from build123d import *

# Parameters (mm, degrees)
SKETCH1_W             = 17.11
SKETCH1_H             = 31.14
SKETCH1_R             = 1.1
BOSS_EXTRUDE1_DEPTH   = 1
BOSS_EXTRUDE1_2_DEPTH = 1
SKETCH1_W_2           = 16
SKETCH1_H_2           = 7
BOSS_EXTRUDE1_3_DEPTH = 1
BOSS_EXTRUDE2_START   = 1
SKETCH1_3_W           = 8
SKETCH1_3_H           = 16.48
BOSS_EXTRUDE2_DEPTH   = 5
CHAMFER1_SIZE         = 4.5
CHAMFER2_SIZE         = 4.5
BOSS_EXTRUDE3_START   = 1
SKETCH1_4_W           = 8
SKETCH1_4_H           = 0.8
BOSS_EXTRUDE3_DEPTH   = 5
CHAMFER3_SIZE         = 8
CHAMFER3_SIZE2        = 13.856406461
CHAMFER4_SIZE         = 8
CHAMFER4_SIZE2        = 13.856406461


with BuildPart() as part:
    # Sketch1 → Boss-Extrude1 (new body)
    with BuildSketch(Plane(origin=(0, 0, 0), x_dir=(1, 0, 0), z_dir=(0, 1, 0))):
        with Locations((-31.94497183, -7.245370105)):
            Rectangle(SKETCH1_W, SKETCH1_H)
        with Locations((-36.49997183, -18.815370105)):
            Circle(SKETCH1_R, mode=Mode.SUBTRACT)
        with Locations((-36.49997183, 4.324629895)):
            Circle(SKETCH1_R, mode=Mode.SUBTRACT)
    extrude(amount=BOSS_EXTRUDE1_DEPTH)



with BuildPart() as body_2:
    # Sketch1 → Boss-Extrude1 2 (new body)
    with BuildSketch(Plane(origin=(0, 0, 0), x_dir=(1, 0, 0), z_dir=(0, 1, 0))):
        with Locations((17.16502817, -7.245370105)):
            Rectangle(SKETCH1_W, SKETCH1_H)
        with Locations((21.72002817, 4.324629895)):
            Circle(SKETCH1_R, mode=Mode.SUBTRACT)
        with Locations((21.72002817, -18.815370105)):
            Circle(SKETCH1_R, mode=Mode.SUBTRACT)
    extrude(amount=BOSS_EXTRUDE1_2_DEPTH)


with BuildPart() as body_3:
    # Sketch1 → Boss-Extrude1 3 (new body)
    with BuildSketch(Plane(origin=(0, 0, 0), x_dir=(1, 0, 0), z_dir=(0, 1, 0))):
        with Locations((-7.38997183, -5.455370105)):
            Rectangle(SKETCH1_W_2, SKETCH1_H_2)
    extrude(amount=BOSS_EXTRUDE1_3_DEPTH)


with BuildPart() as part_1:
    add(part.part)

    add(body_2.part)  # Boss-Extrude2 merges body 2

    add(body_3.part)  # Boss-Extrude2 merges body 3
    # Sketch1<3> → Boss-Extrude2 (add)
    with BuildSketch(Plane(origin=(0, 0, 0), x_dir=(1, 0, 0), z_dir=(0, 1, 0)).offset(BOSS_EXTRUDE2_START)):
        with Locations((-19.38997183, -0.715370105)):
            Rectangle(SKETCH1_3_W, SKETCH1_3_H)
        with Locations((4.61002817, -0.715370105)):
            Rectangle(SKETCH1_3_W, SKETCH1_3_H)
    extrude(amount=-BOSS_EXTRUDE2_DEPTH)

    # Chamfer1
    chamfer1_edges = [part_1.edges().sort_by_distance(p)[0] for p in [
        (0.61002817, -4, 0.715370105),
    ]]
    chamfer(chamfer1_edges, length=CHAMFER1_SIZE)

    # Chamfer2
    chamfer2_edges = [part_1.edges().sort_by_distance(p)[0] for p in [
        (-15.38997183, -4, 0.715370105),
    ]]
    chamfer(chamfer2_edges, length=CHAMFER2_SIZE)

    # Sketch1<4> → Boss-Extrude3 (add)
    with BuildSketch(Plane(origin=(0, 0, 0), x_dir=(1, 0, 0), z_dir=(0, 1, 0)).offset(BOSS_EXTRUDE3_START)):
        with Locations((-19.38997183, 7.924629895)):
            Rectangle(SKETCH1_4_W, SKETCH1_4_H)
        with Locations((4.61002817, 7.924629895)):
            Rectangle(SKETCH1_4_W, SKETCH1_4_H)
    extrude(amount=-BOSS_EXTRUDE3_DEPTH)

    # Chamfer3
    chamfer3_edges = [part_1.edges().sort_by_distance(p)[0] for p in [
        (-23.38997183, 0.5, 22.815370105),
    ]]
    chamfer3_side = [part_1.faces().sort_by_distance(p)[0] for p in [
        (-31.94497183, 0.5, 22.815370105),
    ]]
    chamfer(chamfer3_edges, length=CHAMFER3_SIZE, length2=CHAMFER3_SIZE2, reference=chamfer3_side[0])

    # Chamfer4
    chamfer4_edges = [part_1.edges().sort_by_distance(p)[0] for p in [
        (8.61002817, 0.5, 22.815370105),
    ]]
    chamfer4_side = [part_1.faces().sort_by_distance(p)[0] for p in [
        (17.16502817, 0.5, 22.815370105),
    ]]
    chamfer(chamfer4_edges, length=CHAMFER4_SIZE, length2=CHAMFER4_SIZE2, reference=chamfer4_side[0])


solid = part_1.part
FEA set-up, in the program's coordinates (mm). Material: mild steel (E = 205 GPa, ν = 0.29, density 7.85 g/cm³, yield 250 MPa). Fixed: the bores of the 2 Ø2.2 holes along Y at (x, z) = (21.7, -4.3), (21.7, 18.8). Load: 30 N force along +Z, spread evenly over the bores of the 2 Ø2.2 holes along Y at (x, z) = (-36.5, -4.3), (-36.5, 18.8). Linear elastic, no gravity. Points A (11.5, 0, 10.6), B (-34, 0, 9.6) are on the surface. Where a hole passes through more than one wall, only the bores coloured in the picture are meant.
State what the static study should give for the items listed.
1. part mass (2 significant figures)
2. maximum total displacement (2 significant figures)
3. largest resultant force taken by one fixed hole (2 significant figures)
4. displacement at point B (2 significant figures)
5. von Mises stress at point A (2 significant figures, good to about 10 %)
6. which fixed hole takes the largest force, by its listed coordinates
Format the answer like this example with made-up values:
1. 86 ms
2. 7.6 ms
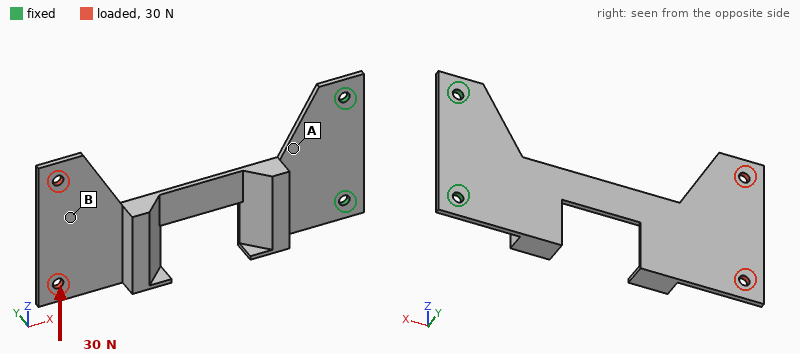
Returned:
1. 17 g
2. 0.14 mm
3. 85 N
4. 0.10 mm
5. 21 MPa
6. (21.7, 18.8)
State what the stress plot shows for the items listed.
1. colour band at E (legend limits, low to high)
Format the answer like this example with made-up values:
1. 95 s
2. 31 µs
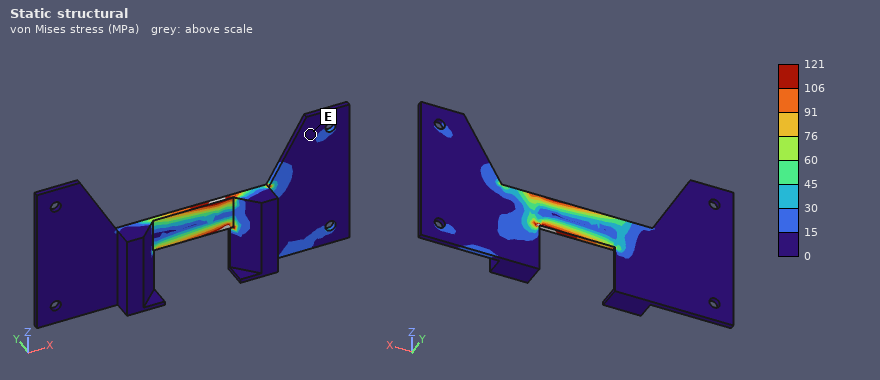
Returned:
1. 0 to 15 MPa
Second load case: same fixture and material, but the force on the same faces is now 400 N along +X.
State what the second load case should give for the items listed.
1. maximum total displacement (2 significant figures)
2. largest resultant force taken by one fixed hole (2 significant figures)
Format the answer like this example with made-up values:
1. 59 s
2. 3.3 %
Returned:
1. 0.15 mm
2. 230 N
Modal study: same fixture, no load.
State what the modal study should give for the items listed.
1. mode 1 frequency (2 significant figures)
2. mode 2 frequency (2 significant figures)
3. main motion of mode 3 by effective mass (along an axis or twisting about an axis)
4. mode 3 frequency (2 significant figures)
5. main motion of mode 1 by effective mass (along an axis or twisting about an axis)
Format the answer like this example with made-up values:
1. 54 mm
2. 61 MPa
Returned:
1. 160 Hz
2. 680 Hz
3. along Y
4. 1100 Hz
5. along Y
